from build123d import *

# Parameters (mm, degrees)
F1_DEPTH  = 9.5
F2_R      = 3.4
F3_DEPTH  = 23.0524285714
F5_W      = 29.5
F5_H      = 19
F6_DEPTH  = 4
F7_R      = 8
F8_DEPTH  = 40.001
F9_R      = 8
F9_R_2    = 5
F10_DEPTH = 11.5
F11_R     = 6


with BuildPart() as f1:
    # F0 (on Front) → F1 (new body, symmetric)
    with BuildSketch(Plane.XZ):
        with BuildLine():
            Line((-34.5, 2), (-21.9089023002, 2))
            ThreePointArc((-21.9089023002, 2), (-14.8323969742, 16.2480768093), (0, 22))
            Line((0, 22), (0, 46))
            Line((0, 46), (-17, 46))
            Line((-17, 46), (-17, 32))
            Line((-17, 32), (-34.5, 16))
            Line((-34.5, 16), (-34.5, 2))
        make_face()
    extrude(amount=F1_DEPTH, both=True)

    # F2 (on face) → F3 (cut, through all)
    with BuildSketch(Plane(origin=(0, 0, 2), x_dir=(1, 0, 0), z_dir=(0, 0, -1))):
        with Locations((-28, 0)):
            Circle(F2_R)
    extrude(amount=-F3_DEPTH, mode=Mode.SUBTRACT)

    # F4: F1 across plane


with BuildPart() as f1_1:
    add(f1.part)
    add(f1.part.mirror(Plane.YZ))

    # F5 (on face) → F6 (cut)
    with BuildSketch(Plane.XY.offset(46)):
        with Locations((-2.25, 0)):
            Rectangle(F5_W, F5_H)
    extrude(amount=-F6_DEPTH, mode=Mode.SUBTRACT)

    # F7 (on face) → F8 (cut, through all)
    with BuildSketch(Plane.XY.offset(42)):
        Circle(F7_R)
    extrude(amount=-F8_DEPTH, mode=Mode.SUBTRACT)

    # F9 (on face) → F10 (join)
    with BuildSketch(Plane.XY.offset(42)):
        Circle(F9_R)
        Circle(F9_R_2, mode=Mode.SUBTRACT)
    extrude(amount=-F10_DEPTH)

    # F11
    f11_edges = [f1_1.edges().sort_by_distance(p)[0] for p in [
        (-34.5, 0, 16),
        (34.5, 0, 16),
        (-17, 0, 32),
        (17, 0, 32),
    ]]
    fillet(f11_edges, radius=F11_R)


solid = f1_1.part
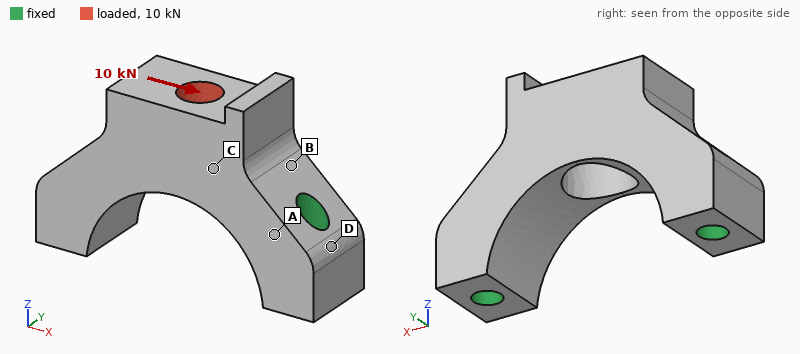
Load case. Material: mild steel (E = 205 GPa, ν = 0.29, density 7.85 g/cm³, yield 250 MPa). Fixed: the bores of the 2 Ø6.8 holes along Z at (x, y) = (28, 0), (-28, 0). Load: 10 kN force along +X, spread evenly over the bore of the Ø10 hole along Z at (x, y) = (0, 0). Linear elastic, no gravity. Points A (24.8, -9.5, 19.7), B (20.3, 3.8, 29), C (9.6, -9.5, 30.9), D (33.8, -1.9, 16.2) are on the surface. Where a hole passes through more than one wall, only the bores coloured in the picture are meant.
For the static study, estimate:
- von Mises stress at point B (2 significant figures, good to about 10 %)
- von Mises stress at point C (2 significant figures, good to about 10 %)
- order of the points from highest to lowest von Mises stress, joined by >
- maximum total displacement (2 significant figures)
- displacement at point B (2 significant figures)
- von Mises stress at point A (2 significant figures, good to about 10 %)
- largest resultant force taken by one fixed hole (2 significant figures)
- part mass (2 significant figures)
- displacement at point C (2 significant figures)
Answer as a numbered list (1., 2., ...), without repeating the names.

1. 44 MPa
2. 33 MPa
3. B > C > A > D
4. 7.3 µm
5. 2.8 µm
6. 18 MPa
7. 6.0 kN
8. 190 g
9. 4.3 µm
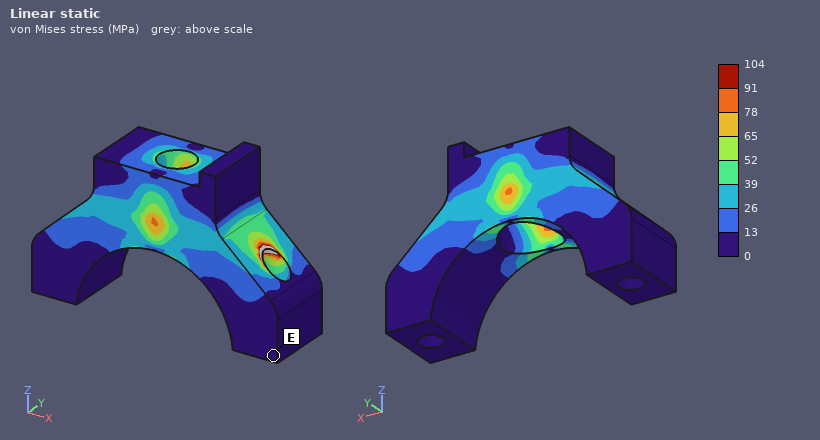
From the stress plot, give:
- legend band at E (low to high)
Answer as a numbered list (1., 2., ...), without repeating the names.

1. 0 to 13 MPa
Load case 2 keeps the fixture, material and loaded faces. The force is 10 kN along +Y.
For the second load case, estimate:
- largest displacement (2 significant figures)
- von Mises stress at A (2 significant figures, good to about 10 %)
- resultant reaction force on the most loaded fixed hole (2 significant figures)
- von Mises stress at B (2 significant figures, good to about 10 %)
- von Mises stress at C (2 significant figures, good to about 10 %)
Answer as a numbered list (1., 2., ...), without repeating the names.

1. 45 µm
2. 110 MPa
3. 5.0 kN
4. 120 MPa
5. 41 MPa
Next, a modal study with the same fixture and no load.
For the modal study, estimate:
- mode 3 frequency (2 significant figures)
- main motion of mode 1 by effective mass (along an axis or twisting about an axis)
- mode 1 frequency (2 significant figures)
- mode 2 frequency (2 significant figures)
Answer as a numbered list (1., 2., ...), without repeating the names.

1. 23 kHz
2. along Y
3. 11 kHz
4. 23 kHz
